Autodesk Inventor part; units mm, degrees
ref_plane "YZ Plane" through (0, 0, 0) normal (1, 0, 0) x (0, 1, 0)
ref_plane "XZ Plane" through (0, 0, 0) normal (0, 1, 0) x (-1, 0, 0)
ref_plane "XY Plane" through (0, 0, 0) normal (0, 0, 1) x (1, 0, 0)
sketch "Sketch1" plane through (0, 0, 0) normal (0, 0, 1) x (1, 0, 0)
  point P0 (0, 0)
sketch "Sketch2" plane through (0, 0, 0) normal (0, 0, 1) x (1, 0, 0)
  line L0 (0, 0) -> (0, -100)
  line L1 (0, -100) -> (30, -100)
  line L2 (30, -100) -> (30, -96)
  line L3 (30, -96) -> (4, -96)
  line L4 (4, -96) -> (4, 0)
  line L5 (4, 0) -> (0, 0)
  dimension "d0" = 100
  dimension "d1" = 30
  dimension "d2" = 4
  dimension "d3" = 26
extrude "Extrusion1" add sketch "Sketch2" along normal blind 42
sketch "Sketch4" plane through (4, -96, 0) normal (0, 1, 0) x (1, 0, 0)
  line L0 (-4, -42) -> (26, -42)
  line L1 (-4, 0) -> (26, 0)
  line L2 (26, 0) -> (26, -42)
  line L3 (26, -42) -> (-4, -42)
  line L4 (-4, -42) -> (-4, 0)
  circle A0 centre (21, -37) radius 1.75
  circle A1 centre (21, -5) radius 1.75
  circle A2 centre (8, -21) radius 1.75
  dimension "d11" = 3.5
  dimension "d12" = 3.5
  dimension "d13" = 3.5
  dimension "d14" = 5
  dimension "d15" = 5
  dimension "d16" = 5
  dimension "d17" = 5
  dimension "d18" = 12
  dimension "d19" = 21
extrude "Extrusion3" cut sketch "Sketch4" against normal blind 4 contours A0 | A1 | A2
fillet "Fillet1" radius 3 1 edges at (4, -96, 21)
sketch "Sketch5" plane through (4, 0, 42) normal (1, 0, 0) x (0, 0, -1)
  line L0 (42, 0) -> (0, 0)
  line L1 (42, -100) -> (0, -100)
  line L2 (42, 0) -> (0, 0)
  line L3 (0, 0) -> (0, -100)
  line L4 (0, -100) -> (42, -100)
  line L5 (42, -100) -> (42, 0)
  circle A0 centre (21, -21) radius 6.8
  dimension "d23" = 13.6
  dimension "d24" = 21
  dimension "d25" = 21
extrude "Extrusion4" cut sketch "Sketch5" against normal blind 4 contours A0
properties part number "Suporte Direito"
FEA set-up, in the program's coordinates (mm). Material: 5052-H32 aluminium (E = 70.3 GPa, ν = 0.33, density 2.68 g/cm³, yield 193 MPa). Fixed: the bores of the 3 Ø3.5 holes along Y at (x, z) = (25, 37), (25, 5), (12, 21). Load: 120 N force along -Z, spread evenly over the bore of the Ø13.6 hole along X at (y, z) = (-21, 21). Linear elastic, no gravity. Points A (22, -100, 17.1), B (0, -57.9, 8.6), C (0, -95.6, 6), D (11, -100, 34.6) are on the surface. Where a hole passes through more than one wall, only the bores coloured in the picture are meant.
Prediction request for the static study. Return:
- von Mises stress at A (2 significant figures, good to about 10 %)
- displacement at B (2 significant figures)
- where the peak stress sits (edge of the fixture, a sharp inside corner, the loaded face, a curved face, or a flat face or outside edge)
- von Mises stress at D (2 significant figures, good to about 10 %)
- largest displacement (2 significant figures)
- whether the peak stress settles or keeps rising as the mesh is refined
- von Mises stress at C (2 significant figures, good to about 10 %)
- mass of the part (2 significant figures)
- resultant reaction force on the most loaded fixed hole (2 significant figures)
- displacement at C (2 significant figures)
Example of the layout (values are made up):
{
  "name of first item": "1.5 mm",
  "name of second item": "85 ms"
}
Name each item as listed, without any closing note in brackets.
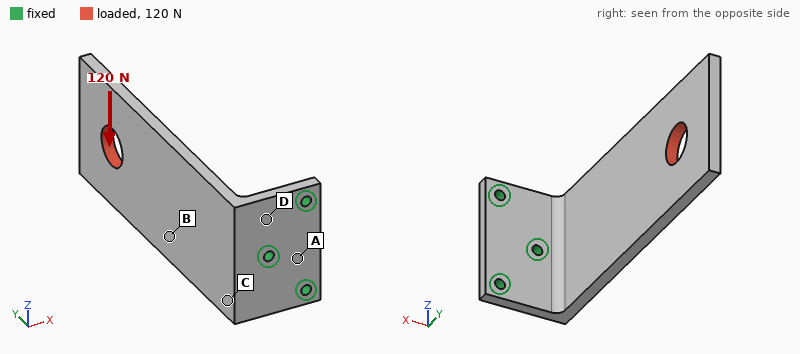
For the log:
{
  "von Mises stress at A": "11 MPa",
  "displacement at B": "0.12 mm",
  "where the peak stress sits": "edge of the fixture",
  "von Mises stress at D": "26 MPa",
  "largest displacement": "0.30 mm",
  "whether the peak stress settles or keeps rising as the mesh is refined": "keeps rising",
  "von Mises stress at C": "22 MPa",
  "mass of the part": "55 g",
  "resultant reaction force on the most loaded fixed hole": "170 N",
  "displacement at C": "0.046 mm"
}
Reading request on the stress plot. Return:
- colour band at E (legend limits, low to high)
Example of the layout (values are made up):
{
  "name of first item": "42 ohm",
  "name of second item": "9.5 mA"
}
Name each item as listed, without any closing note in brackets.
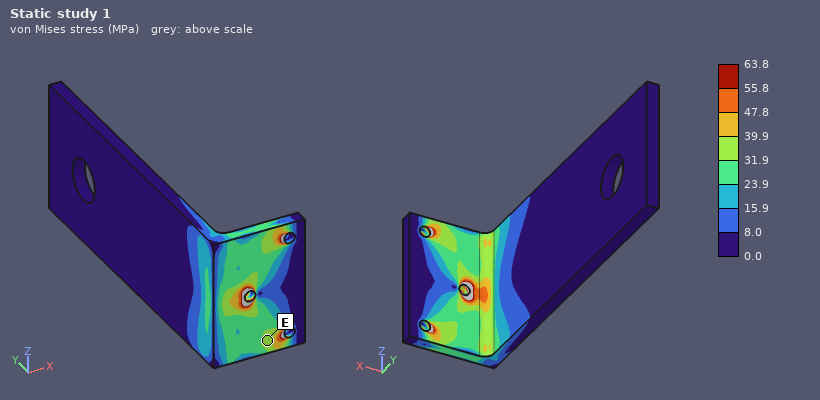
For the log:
{
  "colour band at E": "31.9 to 39.9 MPa"
}
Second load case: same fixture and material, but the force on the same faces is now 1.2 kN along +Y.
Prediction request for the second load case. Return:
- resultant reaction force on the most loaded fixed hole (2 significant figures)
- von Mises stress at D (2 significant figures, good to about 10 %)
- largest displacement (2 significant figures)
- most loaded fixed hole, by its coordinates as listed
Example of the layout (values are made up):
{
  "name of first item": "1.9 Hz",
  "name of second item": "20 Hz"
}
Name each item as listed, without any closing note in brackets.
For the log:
{
  "resultant reaction force on the most loaded fixed hole": "1.5 kN",
  "von Mises stress at D": "40 MPa",
  "largest displacement": "0.51 mm",
  "most loaded fixed hole, by its coordinates as listed": "(12, 21)"
}
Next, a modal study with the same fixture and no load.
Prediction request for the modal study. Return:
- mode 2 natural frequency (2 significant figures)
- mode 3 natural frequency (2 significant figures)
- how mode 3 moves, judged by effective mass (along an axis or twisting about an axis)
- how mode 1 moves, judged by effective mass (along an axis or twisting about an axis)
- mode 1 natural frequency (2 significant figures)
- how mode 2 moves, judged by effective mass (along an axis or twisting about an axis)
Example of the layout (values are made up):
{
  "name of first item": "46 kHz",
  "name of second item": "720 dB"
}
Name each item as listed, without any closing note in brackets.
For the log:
{
  "mode 2 natural frequency": "760 Hz",
  "mode 3 natural frequency": "1600 Hz",
  "how mode 3 moves, judged by effective mass": "twisting about Y",
  "how mode 1 moves, judged by effective mass": "along X",
  "mode 1 natural frequency": "320 Hz",
  "how mode 2 moves, judged by effective mass": "along Z"
}
